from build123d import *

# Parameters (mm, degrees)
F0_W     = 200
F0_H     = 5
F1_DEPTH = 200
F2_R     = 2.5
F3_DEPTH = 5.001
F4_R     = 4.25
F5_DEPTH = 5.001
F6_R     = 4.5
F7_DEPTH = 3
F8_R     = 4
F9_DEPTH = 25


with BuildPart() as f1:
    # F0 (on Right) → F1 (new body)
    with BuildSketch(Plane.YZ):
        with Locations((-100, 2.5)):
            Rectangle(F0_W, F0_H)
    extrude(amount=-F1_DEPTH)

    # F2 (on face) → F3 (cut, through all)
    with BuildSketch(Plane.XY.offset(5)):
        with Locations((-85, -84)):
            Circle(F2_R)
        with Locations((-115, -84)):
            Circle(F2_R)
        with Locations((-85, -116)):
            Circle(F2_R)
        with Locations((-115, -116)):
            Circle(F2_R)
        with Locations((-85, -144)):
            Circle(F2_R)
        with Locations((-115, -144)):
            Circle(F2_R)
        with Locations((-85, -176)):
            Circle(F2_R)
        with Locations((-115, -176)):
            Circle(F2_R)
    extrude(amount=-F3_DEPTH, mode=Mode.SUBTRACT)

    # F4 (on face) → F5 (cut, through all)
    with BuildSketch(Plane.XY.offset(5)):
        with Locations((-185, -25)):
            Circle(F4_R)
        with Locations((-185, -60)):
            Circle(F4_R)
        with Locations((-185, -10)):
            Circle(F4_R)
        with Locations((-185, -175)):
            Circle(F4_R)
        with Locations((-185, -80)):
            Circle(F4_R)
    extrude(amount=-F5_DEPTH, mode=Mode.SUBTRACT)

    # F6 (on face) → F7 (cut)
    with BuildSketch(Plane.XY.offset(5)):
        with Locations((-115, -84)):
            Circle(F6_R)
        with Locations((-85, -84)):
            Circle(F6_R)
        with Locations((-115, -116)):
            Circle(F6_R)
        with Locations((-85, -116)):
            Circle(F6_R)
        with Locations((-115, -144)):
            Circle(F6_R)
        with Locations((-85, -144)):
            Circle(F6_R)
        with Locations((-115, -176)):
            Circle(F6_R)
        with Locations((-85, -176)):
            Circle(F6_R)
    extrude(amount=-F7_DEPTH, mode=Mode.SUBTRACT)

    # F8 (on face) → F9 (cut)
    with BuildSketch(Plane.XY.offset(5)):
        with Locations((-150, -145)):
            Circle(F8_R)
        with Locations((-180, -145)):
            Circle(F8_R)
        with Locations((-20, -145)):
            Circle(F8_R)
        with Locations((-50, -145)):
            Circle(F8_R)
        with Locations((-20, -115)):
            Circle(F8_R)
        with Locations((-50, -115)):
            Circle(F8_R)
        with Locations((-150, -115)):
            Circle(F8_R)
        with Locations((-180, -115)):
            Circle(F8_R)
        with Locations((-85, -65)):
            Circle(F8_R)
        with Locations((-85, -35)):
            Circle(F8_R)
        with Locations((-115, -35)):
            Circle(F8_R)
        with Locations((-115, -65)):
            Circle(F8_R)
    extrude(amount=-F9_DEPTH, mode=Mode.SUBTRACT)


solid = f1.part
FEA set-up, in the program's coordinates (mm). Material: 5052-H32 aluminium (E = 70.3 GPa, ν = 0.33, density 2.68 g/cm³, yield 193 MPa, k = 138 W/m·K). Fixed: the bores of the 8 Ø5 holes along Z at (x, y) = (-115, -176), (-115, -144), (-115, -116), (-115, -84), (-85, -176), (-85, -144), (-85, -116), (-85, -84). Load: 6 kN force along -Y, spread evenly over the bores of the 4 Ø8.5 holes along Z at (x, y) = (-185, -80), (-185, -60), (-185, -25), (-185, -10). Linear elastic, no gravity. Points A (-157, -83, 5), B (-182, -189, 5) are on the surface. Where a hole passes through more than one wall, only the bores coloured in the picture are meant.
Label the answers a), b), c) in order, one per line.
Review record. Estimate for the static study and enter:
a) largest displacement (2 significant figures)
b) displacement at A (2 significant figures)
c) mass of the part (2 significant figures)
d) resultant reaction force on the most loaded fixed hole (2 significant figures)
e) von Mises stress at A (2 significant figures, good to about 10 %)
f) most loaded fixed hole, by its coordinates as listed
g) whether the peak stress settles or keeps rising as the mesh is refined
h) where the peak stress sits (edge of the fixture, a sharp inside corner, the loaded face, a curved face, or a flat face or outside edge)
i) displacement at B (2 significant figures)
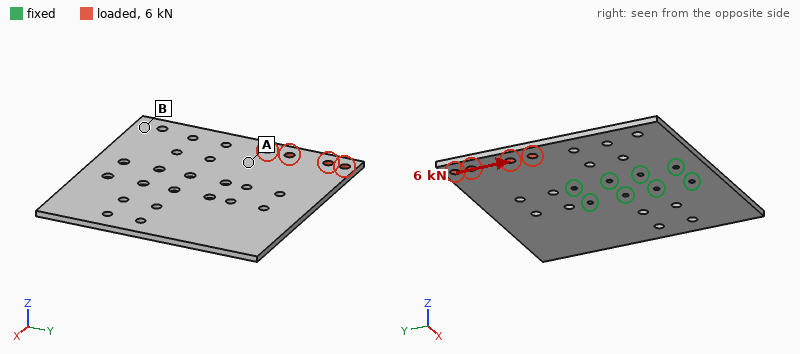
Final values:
a) 92 µm
b) 33 µm
c) 520 g
d) 3.3 kN
e) 18 MPa
f) (-115, -84)
g) keeps rising
h) edge of the fixture
i) 39 µm
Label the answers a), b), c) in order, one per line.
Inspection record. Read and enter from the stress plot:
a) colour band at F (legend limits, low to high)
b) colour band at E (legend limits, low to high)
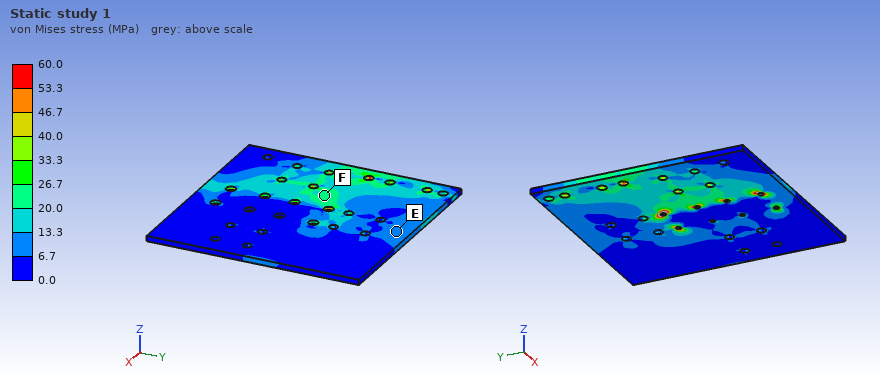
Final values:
a) 20.0 to 26.7 MPa
b) 6.7 to 13.3 MPa
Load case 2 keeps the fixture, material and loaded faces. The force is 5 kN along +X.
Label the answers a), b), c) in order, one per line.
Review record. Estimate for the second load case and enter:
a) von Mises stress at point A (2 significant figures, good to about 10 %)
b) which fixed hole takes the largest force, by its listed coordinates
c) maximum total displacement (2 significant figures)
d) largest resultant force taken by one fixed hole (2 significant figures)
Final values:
a) 13 MPa
b) (-115, -84)
c) 82 µm
d) 3.1 kN
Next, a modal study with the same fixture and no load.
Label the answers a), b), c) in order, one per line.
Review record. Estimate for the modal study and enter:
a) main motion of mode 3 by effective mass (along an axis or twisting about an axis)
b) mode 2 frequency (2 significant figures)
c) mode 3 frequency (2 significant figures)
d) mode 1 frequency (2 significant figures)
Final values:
a) along Z
b) 400 Hz
c) 540 Hz
d) 390 Hz
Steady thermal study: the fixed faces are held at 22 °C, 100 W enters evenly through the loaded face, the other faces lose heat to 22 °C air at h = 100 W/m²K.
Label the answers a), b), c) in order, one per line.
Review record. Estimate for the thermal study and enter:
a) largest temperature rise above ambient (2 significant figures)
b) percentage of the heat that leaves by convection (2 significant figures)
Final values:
a) 73 K
b) 78 %
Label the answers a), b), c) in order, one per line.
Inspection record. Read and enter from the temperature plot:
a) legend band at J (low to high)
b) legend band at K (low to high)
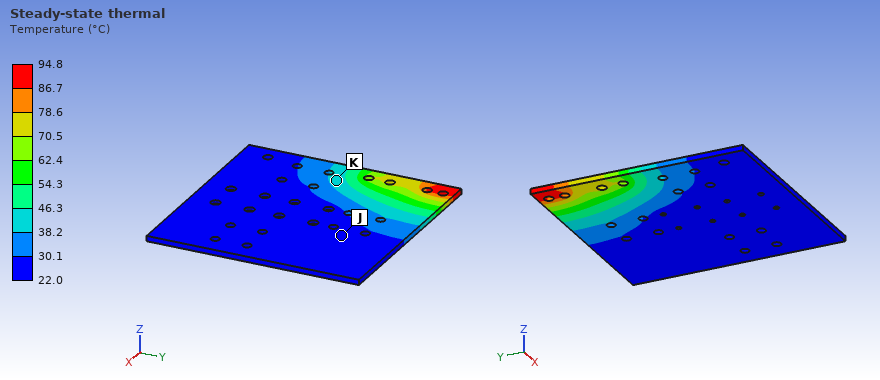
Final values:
a) 22.0 to 30.1 °C
b) 38.2 to 46.3 °C
